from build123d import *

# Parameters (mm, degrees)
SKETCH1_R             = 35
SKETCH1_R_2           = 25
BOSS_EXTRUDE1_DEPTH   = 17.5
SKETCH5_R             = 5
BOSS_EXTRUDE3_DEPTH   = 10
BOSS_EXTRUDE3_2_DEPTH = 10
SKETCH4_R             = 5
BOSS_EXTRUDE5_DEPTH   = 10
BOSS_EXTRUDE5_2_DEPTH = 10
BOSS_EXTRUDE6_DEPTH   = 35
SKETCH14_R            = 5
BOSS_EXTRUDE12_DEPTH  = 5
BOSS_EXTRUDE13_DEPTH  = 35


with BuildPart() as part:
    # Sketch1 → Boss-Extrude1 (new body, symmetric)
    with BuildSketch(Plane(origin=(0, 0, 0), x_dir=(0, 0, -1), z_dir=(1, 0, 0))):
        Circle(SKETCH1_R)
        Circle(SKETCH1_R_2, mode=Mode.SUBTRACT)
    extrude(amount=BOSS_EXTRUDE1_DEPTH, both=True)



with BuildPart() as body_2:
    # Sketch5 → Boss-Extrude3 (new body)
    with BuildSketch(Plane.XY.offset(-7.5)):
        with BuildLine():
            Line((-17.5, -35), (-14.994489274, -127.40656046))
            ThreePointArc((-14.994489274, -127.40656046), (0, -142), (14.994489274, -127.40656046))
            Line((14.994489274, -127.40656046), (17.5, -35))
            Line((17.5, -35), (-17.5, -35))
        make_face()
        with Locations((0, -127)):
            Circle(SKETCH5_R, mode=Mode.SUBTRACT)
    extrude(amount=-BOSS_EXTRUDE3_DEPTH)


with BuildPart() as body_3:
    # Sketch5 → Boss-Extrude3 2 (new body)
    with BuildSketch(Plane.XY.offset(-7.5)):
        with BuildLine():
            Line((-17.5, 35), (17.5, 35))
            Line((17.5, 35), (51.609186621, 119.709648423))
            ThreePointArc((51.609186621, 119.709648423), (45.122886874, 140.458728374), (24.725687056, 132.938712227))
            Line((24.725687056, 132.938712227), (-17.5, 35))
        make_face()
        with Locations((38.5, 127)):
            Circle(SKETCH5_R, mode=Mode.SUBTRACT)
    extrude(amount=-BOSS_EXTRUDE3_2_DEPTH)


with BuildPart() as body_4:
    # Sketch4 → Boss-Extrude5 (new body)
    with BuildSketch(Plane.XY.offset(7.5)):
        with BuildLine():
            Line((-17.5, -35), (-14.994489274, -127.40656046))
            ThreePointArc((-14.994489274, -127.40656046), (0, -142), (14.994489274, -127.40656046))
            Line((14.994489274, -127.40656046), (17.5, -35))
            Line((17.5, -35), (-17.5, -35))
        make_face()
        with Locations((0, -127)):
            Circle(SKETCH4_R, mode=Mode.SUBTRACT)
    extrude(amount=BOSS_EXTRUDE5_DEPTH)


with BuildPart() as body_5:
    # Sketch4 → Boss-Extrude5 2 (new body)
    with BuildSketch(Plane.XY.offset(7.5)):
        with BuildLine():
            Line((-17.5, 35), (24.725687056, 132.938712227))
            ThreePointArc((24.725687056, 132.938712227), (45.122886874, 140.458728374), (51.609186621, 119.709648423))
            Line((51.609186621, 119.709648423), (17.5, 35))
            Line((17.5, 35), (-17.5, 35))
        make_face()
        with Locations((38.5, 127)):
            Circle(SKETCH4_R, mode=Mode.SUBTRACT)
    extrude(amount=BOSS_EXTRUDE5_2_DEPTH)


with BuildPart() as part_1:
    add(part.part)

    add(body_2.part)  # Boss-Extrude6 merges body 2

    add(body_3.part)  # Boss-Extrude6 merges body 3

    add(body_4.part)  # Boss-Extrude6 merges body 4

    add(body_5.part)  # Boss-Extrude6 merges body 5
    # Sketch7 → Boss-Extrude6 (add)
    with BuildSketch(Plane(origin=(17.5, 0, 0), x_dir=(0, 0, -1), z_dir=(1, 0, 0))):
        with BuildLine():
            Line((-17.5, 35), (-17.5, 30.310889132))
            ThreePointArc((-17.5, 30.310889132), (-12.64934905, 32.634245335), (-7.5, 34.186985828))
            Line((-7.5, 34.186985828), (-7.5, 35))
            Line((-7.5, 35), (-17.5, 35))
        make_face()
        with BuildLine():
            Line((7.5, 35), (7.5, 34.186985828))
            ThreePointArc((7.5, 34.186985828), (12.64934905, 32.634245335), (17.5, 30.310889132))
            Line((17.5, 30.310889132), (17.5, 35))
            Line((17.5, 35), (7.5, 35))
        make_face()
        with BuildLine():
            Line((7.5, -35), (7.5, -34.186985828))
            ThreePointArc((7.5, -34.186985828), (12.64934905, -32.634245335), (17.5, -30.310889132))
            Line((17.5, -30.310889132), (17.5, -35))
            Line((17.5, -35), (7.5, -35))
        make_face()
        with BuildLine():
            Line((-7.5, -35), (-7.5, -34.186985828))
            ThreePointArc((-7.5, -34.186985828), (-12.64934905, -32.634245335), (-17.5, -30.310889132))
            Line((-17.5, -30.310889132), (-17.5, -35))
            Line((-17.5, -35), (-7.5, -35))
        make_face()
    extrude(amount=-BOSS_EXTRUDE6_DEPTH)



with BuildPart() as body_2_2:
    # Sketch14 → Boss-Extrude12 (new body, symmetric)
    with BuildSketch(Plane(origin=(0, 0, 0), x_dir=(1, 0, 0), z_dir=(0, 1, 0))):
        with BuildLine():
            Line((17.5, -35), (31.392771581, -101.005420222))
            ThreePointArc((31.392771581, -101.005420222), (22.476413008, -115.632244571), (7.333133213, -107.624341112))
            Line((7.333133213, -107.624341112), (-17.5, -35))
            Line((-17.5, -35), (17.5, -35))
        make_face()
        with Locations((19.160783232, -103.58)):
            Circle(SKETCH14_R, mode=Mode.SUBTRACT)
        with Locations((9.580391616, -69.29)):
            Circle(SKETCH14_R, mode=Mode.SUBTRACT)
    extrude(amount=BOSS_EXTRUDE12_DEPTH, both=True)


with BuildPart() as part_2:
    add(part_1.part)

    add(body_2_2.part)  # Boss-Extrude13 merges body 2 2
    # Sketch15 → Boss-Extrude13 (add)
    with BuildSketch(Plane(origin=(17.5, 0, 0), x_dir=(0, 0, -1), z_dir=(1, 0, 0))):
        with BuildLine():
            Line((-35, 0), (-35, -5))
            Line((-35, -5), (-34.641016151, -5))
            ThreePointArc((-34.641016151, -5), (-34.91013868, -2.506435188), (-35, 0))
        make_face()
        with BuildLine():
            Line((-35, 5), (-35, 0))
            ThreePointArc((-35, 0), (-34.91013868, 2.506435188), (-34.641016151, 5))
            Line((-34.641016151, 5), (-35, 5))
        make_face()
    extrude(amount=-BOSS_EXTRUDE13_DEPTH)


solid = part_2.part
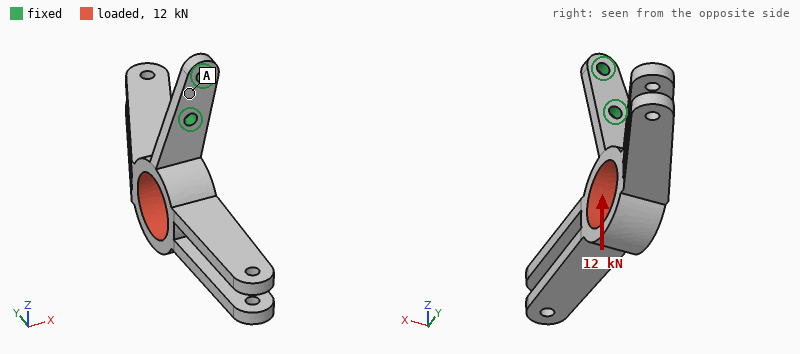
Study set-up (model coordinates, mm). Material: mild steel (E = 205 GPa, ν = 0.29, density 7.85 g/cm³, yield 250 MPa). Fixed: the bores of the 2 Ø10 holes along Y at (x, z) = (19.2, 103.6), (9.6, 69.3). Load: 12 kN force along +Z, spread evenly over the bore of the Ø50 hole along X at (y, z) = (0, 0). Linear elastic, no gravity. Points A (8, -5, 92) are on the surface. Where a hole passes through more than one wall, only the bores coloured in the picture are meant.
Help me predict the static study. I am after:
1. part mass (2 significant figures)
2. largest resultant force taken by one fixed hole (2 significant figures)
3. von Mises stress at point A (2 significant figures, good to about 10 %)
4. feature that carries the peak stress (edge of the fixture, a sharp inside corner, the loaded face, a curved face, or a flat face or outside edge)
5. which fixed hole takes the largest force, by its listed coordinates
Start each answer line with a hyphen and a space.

- 1.8 kg
- 12 kN
- 16 MPa
- edge of the fixture
- (9.6, 69.3)
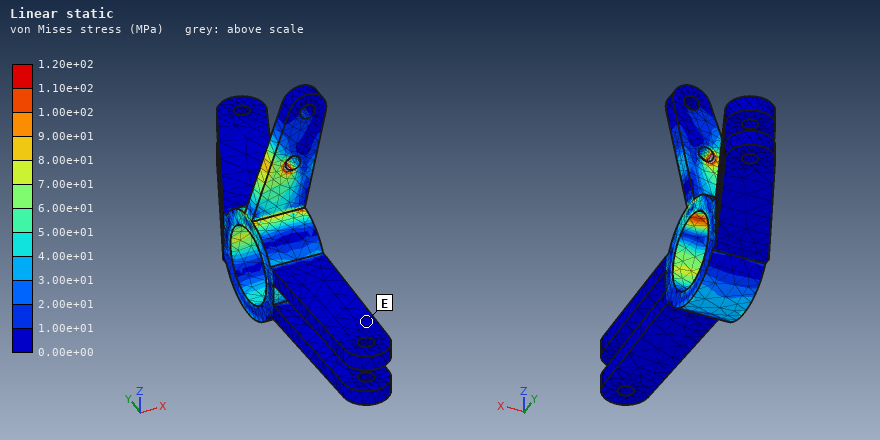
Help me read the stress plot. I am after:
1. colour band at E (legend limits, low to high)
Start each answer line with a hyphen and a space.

- 0.00e+00 to 1.00e+01 MPa
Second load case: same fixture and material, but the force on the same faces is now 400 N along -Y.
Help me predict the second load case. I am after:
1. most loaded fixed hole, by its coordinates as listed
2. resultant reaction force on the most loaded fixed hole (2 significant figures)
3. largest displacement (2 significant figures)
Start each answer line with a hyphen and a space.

- (9.6, 69.3)
- 480 N
- 0.23 mm
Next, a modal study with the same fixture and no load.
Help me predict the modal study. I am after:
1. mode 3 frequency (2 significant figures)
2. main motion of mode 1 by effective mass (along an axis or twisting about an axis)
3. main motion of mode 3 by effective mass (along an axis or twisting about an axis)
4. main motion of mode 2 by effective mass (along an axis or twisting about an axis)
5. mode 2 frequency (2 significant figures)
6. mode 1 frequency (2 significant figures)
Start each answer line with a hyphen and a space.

- 600 Hz
- along Y
- along X
- twisting about Z
- 250 Hz
- 160 Hz
